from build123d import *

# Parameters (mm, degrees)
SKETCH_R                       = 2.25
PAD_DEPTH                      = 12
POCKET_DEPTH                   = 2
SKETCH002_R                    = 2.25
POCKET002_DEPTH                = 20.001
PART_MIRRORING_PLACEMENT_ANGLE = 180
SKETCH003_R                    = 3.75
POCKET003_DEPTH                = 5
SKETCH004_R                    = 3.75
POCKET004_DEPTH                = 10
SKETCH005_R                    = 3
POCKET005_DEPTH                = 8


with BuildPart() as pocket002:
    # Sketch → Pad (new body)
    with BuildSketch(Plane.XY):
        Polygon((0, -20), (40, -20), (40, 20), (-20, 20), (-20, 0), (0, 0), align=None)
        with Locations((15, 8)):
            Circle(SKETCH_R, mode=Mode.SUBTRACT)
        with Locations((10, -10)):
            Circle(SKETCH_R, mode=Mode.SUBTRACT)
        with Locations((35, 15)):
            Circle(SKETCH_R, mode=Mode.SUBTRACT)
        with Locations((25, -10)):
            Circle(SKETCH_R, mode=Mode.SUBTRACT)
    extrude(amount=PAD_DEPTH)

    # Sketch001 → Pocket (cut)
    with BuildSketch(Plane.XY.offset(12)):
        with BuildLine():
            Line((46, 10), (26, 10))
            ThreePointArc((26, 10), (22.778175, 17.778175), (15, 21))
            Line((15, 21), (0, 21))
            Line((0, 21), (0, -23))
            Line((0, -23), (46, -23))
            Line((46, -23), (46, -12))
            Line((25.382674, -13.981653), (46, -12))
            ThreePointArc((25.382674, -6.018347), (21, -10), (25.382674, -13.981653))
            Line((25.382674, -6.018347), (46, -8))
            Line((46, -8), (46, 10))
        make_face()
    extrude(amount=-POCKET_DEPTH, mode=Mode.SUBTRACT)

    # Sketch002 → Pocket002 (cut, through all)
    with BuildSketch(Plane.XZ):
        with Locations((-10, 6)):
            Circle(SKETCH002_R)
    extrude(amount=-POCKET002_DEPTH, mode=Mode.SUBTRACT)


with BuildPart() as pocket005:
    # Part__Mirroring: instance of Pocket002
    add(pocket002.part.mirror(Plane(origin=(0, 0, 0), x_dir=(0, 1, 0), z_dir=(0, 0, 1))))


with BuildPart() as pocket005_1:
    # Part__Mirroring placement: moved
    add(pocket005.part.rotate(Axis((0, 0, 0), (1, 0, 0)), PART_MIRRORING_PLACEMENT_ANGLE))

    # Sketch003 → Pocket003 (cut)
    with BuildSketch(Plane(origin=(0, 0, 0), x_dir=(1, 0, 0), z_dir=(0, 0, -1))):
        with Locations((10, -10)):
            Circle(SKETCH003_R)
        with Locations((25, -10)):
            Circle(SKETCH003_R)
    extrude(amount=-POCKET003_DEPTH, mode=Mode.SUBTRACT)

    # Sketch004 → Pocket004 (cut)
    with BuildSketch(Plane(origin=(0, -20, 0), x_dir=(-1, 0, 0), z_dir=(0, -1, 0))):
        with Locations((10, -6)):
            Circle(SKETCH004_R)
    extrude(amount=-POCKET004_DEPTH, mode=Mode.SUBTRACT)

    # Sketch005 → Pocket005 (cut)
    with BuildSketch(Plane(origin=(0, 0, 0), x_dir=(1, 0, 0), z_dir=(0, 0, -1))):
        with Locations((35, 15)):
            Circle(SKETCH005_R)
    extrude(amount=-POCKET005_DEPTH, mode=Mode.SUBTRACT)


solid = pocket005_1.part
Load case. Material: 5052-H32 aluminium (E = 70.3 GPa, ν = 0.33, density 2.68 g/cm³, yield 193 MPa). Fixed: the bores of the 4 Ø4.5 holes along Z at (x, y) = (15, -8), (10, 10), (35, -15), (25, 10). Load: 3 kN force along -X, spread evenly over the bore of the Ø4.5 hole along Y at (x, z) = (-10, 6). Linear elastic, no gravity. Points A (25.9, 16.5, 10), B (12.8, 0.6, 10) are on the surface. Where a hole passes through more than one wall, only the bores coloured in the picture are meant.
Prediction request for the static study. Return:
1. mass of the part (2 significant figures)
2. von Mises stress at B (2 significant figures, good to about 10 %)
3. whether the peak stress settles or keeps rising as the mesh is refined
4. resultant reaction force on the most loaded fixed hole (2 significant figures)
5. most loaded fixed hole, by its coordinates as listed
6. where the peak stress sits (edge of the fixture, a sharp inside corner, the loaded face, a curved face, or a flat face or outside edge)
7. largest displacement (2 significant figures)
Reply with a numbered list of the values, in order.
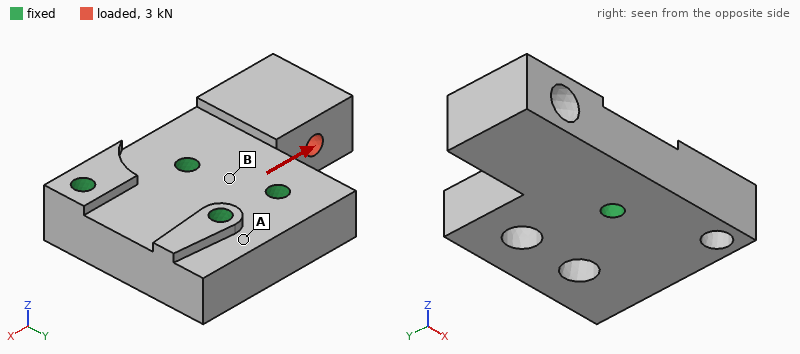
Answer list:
1. 53 g
2. 9.6 MPa
3. keeps rising
4. 2.2 kN
5. (15, -8)
6. a sharp inside corner
7. 17 µm
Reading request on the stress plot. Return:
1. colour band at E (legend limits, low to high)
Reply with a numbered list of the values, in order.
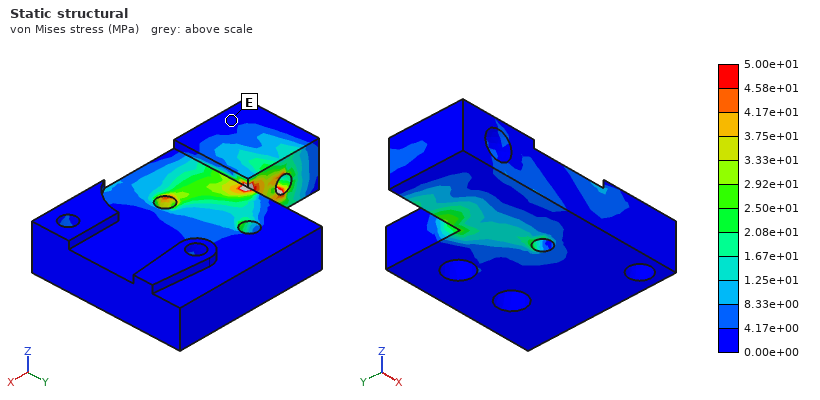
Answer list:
1. 0.00e+00 to 4.17e+00 MPa
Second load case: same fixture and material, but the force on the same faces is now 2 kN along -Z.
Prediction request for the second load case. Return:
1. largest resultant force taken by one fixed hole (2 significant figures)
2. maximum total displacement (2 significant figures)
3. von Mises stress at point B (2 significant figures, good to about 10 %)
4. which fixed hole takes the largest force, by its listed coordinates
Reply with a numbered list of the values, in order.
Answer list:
1. 2.0 kN
2. 0.13 mm
3. 46 MPa
4. (15, -8)
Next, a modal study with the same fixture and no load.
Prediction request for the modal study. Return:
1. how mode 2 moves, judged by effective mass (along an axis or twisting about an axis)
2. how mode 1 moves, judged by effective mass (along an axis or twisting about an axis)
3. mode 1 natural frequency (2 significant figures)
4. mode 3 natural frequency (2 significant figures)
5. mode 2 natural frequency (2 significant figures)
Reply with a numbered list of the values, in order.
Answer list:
1. along Y
2. along Z
3. 6700 Hz
4. 19 kHz
5. 13 kHz
